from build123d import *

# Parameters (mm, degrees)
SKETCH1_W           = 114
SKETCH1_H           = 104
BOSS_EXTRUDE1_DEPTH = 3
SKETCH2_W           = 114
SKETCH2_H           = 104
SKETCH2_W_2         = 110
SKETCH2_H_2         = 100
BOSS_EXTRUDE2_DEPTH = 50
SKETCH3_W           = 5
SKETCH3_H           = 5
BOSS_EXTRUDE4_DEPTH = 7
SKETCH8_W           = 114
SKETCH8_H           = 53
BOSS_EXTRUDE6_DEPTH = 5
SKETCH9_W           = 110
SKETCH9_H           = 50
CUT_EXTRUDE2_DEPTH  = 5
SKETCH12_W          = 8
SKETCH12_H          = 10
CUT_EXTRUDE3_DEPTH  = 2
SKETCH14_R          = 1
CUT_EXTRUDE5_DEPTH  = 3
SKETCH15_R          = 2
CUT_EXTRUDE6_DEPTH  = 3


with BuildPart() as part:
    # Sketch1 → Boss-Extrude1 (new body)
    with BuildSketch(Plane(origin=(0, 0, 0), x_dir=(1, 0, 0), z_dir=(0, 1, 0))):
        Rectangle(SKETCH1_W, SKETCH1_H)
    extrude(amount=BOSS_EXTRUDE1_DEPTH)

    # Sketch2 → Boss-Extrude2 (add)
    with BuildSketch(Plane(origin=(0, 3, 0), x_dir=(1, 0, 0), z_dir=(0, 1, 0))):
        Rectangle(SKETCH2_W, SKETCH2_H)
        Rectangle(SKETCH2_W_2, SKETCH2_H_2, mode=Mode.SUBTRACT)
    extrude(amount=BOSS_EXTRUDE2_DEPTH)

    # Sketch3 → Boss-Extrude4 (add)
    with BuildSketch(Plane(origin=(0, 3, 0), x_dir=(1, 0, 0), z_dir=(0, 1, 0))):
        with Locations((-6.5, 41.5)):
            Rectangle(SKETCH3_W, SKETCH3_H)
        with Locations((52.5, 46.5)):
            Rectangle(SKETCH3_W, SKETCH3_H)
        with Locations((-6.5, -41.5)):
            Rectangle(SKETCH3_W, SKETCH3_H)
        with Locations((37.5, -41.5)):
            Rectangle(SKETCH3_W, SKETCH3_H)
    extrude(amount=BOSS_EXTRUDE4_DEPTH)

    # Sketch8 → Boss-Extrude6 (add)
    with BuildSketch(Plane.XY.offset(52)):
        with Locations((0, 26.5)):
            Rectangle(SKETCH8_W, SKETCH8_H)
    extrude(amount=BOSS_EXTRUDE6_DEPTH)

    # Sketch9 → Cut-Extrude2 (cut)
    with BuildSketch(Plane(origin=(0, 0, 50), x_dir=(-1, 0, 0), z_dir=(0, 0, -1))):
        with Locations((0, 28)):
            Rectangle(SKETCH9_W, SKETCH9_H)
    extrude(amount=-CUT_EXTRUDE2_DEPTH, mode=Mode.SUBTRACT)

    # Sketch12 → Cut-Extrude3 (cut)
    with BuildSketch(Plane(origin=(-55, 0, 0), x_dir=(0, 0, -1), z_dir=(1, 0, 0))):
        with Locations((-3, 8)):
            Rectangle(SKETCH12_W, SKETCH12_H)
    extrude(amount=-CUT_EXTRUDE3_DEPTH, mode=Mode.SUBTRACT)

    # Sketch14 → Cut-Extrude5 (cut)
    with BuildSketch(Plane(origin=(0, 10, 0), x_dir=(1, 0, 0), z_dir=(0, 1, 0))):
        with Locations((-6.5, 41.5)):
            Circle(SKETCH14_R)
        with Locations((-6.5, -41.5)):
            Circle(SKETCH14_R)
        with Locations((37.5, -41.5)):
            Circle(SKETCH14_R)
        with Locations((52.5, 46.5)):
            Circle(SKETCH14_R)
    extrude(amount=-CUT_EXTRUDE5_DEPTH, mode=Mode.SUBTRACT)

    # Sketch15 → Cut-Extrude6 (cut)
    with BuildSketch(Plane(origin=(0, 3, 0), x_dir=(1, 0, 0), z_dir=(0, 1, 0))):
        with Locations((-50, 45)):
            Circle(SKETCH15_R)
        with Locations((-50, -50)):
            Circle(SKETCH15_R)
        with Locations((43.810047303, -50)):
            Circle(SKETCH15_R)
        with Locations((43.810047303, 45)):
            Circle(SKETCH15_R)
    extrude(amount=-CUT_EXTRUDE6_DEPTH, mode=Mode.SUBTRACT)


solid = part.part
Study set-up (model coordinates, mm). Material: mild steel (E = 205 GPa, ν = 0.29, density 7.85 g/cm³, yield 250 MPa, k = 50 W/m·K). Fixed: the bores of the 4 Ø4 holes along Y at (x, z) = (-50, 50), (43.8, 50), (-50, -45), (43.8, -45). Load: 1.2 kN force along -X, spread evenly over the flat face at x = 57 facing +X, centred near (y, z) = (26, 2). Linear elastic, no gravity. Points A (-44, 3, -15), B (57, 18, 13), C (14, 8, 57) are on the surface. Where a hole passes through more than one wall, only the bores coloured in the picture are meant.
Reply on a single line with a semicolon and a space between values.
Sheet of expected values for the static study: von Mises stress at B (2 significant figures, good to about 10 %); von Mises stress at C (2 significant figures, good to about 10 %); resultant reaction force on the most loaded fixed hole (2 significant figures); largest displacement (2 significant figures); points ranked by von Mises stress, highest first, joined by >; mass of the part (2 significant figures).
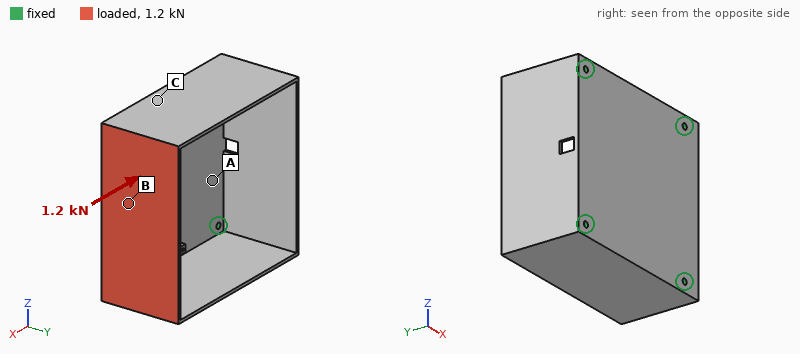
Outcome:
47 MPa; 27 MPa; 360 N; 0.50 mm; B > C > A; 640 g
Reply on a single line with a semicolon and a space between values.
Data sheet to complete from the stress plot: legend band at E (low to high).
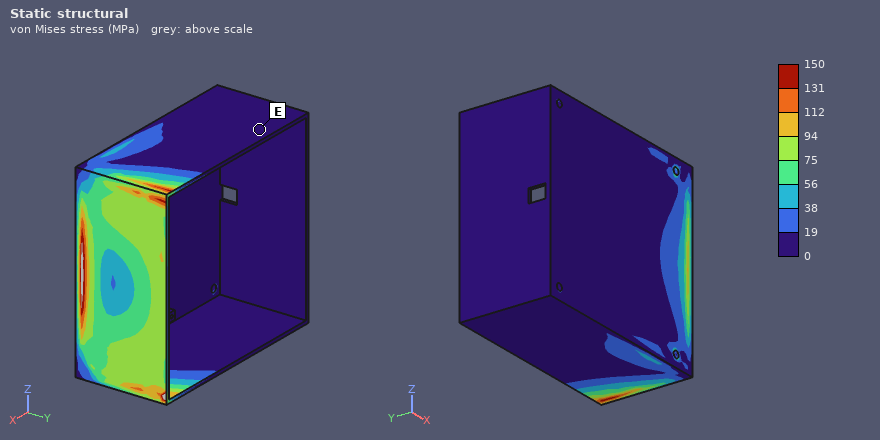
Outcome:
0 to 19 MPa
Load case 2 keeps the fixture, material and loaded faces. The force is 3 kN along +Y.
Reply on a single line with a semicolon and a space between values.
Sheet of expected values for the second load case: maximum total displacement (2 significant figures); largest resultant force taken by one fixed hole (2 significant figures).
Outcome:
89 µm; 1.7 kN
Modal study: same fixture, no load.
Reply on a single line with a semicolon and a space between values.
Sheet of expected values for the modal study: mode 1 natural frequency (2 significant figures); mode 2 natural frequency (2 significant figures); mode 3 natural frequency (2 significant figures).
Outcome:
960 Hz; 1100 Hz; 1100 Hz
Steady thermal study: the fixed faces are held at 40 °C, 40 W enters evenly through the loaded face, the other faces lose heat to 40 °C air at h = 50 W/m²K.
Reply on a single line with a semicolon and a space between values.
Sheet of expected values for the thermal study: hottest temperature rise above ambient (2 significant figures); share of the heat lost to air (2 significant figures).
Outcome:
60 K; 70 %
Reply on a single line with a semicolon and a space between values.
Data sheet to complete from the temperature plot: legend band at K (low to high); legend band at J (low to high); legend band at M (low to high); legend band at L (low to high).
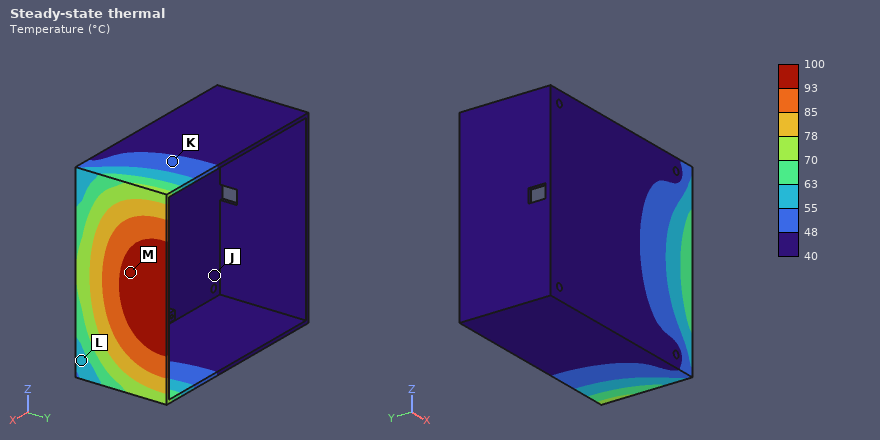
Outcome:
48 to 55 °C; 40 to 48 °C; 93 to 100 °C; 55 to 63 °C
